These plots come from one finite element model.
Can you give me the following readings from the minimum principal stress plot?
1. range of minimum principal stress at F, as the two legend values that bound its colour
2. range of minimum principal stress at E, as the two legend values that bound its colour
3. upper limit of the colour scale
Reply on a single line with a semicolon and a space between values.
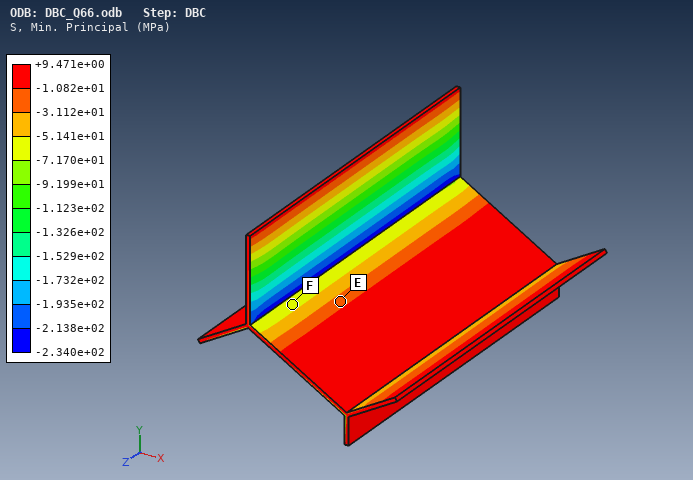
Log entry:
-7.170e+01 to -5.141e+01 MPa; -3.112e+01 to -1.082e+01 MPa; +9.471e+00 MPa
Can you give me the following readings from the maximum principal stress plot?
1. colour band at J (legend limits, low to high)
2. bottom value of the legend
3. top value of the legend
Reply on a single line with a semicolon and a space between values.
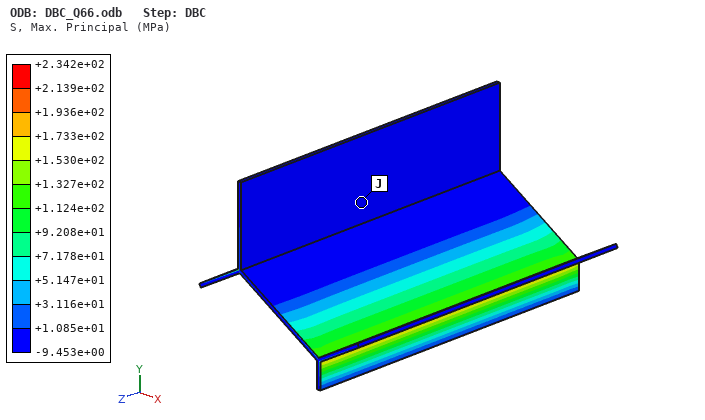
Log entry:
-9.453e+00 to +1.085e+01 MPa; -9.453e+00 MPa; +2.342e+02 MPa
